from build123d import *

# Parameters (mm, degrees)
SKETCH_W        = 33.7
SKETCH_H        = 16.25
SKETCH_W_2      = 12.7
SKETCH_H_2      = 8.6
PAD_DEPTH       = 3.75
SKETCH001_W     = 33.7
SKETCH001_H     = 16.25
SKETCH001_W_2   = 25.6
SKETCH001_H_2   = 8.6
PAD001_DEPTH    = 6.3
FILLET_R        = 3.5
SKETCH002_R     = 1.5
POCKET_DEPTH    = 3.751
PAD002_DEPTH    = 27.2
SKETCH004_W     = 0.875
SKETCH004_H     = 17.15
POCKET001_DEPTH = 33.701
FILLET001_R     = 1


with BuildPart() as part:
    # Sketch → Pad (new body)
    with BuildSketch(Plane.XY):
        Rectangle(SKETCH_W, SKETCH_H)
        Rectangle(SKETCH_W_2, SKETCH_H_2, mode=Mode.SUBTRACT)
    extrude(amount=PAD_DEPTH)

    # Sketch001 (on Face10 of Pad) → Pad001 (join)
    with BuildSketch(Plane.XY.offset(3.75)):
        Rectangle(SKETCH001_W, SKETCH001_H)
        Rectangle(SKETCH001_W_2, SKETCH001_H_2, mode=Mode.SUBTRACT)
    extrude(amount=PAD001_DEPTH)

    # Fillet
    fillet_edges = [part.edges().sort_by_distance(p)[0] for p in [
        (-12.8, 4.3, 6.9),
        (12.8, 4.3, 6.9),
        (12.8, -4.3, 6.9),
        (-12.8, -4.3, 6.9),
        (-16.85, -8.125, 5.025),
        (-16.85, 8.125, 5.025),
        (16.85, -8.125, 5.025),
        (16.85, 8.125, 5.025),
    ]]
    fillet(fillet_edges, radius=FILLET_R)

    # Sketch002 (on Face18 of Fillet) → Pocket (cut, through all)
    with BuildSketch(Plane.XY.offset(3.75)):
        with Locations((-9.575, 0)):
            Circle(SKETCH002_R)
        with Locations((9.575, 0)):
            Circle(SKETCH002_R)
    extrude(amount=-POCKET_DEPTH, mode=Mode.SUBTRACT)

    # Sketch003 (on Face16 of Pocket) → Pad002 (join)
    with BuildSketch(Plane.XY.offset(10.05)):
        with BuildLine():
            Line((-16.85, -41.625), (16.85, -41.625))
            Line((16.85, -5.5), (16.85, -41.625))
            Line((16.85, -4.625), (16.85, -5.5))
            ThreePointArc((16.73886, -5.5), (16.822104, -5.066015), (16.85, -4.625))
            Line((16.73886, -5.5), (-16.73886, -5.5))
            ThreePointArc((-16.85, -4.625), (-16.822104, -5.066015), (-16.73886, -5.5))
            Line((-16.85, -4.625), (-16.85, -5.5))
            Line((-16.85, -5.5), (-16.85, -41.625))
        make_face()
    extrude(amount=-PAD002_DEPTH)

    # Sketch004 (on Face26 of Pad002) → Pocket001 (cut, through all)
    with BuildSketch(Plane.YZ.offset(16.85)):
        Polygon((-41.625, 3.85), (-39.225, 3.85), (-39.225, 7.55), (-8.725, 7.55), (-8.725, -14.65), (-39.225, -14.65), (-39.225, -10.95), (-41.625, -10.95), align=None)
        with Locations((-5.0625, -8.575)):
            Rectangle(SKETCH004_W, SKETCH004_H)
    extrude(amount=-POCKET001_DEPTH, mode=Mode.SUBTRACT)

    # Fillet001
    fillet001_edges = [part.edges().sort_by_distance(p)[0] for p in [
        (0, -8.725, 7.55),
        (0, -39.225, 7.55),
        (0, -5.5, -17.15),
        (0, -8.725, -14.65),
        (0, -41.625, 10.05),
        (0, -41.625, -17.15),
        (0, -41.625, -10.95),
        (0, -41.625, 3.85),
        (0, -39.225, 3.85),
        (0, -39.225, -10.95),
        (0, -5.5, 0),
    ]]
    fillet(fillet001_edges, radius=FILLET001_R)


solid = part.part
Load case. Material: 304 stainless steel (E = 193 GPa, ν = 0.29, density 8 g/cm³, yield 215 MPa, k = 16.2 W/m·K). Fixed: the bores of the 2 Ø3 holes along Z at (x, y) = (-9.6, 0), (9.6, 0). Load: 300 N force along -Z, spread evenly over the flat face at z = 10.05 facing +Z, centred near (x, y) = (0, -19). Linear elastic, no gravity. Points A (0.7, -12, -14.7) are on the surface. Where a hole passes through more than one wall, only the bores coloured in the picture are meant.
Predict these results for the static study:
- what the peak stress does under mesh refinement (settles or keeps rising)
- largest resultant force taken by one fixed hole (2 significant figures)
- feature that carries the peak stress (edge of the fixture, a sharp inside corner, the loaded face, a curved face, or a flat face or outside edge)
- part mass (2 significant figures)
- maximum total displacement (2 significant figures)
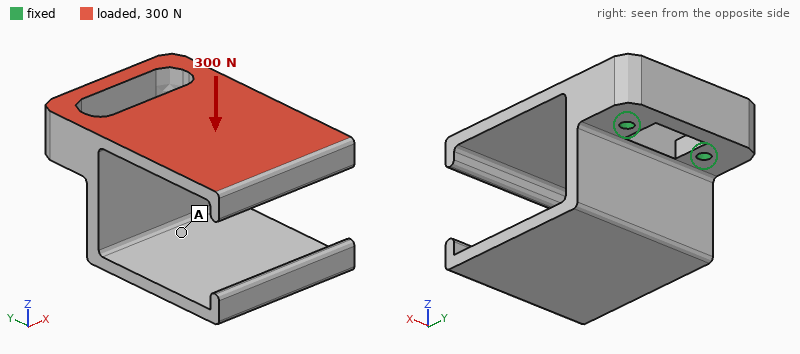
keeps rising
150 N
edge of the fixture
95 g
0.15 mm
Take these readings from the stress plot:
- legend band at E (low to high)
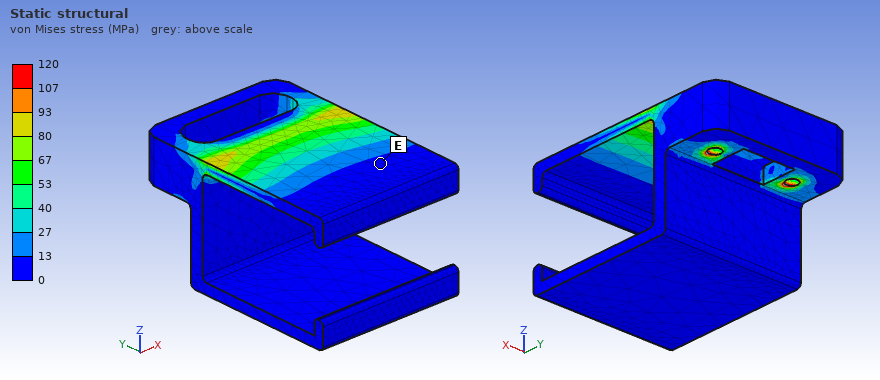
0 to 13 MPa
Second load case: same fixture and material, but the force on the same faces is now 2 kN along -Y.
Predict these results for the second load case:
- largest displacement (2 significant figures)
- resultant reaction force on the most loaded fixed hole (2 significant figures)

0.17 mm
1.0 kN
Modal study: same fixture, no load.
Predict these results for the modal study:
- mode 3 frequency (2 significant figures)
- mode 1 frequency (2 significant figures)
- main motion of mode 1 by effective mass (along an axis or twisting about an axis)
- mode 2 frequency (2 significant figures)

2300 Hz
1000 Hz
along Z
1400 Hz
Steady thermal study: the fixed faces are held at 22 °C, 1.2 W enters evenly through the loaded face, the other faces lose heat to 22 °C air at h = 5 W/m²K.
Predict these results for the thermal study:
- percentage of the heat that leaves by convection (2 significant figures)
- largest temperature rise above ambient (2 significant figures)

15 %
15 K
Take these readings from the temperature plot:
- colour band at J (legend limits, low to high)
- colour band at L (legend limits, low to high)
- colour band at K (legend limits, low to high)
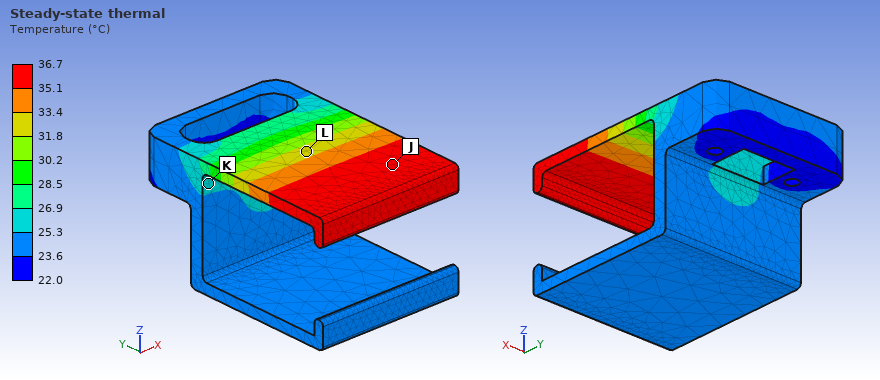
35.1 to 36.7 °C
31.8 to 33.4 °C
25.3 to 26.9 °C
